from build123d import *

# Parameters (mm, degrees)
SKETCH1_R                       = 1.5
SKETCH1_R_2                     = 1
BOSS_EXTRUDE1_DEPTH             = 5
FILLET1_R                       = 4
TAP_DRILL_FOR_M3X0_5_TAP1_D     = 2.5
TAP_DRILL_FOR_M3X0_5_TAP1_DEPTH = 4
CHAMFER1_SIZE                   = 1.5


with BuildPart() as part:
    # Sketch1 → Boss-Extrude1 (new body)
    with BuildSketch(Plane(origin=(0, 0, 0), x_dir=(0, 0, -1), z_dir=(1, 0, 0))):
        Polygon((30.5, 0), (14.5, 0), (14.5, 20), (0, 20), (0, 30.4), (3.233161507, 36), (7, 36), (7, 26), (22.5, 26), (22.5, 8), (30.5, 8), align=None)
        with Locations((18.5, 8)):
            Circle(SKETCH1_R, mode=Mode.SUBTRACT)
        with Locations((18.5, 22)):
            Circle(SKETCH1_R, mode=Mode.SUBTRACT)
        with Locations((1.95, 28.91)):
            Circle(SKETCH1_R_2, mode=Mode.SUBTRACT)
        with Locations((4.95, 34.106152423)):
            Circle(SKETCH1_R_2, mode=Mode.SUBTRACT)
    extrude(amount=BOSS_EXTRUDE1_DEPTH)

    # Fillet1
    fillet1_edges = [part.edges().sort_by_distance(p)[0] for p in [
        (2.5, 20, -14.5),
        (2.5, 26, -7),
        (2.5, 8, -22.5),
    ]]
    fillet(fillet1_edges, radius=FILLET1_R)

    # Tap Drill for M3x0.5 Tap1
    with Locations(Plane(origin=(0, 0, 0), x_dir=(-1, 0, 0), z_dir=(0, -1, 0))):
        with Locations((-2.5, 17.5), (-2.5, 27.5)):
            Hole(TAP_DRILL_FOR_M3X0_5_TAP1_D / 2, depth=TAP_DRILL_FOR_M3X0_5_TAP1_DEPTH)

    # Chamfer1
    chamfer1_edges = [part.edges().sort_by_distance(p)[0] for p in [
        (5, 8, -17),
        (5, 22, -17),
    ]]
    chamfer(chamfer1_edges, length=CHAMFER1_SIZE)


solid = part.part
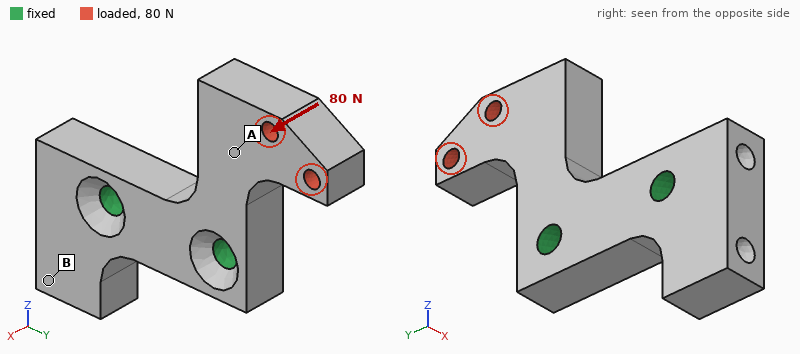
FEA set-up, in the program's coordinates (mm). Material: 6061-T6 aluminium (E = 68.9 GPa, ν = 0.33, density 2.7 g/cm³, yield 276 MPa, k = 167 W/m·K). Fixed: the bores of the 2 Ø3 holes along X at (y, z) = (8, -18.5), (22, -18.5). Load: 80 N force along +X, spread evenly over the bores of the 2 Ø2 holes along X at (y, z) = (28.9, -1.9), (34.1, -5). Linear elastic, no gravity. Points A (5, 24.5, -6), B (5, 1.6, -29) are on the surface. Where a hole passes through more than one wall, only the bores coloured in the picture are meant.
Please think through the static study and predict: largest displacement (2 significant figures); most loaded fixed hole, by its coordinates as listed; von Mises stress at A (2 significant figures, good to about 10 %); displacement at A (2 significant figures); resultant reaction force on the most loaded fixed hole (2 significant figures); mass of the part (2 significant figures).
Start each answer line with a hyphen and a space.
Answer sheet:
- 51 µm
- (22, -18.5)
- 18 MPa
- 20 µm
- 110 N
- 5.4 g
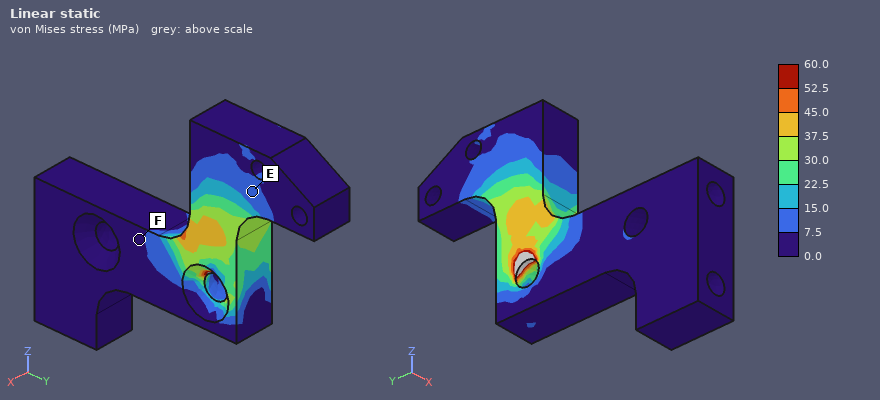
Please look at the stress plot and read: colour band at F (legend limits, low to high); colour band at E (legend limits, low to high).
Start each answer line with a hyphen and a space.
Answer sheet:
- 0.0 to 7.5 MPa
- 7.5 to 15.0 MPa
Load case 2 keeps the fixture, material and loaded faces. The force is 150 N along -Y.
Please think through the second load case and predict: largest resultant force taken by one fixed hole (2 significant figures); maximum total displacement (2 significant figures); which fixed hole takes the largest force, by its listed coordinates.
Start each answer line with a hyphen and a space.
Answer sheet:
- 140 N
- 32 µm
- (8, -18.5)
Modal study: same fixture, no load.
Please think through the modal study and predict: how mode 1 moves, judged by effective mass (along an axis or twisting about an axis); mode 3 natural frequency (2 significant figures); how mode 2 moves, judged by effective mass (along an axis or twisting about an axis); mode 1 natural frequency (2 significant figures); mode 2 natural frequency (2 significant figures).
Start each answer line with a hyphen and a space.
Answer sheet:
- along X
- 17 kHz
- along Y
- 7500 Hz
- 10 kHz
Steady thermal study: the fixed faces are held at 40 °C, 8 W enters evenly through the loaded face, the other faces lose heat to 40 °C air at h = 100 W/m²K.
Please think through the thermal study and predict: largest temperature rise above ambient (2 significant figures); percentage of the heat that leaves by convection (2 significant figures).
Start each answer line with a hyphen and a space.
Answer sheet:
- 27 K
- 12 %
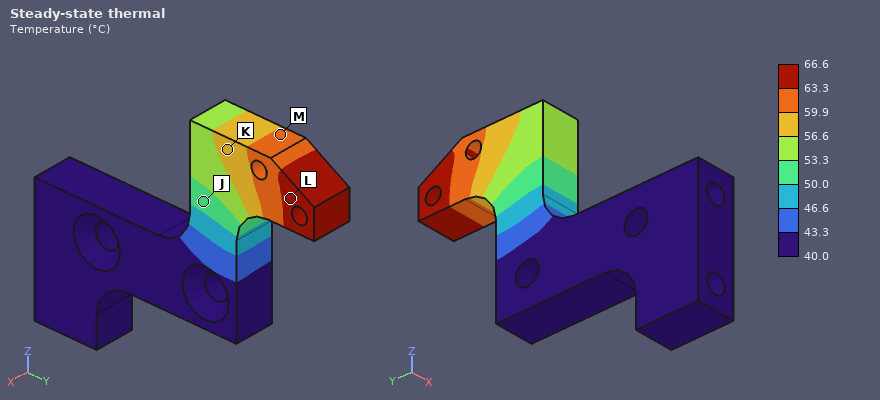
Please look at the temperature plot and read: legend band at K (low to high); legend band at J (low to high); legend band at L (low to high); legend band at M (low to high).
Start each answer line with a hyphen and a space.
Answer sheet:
- 56.6 to 59.9 °C
- 50.0 to 53.3 °C
- 63.3 to 66.6 °C
- 59.9 to 63.3 °C
